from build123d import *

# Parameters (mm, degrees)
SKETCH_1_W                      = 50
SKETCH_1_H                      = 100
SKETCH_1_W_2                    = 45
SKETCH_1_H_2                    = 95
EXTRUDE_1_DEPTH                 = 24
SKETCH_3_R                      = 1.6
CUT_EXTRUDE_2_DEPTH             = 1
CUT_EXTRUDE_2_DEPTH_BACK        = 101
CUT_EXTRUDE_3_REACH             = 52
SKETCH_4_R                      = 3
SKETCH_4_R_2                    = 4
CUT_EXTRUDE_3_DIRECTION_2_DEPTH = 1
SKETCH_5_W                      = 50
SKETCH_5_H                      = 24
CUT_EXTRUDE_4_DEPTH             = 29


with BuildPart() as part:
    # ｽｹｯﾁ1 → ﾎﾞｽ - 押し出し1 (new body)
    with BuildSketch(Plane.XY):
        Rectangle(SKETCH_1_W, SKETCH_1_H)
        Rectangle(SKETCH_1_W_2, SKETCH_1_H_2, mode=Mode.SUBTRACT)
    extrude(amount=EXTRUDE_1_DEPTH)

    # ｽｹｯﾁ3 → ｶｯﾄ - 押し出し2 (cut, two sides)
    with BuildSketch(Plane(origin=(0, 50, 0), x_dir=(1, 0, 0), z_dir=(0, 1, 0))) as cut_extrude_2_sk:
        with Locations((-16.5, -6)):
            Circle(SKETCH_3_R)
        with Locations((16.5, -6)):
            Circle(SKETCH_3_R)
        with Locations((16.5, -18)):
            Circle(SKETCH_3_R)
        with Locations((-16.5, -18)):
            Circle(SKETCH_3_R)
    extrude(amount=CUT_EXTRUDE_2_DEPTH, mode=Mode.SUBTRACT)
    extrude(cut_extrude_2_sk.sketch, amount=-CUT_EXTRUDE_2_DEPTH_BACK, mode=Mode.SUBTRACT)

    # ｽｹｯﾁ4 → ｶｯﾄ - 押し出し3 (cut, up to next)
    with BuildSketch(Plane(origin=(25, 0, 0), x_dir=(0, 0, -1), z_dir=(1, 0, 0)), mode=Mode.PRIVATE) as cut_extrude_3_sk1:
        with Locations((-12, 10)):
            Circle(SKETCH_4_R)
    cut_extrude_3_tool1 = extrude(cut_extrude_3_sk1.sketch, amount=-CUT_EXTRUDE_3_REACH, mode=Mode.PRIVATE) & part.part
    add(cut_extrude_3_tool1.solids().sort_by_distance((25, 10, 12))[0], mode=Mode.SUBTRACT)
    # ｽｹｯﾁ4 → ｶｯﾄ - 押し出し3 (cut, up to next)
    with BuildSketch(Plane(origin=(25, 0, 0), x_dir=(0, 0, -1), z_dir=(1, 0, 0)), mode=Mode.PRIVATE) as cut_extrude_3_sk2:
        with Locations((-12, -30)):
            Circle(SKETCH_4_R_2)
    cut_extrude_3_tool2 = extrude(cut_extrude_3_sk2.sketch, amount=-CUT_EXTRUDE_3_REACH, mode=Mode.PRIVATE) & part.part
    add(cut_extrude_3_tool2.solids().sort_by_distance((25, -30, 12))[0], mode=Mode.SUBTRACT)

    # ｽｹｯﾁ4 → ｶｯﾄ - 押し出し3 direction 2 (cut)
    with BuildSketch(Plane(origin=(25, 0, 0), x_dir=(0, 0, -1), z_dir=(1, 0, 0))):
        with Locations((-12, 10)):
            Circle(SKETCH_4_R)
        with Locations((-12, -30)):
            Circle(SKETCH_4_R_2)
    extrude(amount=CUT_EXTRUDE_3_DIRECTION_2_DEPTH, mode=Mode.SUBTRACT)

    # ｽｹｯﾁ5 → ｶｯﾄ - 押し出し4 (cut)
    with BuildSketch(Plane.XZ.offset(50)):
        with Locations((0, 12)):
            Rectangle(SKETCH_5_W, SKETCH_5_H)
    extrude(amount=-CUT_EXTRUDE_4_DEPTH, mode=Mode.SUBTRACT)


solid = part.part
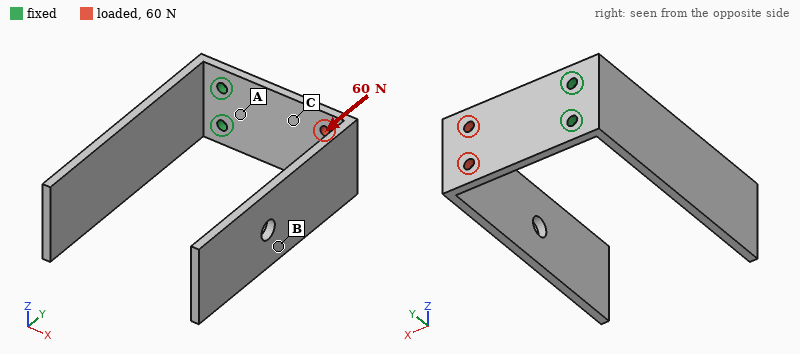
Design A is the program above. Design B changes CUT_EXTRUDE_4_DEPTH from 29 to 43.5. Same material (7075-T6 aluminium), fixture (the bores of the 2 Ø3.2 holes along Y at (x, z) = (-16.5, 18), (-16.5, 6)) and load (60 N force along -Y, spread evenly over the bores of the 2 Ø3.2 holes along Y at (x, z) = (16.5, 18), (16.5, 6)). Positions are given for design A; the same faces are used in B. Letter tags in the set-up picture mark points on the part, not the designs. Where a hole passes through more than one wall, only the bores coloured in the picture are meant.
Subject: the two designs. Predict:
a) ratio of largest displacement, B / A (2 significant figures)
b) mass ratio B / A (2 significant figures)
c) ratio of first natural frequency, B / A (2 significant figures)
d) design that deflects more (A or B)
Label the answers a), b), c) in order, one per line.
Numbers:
a) 0.83
b) 0.84
c) 1.4
d) A
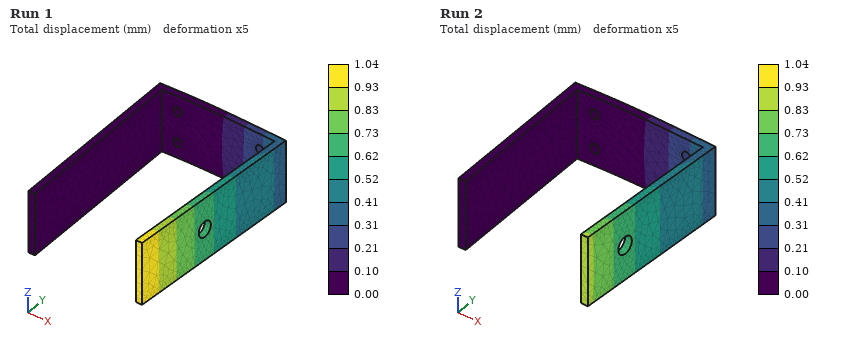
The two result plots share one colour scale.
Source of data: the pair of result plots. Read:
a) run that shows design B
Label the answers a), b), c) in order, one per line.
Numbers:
a) Run 2
